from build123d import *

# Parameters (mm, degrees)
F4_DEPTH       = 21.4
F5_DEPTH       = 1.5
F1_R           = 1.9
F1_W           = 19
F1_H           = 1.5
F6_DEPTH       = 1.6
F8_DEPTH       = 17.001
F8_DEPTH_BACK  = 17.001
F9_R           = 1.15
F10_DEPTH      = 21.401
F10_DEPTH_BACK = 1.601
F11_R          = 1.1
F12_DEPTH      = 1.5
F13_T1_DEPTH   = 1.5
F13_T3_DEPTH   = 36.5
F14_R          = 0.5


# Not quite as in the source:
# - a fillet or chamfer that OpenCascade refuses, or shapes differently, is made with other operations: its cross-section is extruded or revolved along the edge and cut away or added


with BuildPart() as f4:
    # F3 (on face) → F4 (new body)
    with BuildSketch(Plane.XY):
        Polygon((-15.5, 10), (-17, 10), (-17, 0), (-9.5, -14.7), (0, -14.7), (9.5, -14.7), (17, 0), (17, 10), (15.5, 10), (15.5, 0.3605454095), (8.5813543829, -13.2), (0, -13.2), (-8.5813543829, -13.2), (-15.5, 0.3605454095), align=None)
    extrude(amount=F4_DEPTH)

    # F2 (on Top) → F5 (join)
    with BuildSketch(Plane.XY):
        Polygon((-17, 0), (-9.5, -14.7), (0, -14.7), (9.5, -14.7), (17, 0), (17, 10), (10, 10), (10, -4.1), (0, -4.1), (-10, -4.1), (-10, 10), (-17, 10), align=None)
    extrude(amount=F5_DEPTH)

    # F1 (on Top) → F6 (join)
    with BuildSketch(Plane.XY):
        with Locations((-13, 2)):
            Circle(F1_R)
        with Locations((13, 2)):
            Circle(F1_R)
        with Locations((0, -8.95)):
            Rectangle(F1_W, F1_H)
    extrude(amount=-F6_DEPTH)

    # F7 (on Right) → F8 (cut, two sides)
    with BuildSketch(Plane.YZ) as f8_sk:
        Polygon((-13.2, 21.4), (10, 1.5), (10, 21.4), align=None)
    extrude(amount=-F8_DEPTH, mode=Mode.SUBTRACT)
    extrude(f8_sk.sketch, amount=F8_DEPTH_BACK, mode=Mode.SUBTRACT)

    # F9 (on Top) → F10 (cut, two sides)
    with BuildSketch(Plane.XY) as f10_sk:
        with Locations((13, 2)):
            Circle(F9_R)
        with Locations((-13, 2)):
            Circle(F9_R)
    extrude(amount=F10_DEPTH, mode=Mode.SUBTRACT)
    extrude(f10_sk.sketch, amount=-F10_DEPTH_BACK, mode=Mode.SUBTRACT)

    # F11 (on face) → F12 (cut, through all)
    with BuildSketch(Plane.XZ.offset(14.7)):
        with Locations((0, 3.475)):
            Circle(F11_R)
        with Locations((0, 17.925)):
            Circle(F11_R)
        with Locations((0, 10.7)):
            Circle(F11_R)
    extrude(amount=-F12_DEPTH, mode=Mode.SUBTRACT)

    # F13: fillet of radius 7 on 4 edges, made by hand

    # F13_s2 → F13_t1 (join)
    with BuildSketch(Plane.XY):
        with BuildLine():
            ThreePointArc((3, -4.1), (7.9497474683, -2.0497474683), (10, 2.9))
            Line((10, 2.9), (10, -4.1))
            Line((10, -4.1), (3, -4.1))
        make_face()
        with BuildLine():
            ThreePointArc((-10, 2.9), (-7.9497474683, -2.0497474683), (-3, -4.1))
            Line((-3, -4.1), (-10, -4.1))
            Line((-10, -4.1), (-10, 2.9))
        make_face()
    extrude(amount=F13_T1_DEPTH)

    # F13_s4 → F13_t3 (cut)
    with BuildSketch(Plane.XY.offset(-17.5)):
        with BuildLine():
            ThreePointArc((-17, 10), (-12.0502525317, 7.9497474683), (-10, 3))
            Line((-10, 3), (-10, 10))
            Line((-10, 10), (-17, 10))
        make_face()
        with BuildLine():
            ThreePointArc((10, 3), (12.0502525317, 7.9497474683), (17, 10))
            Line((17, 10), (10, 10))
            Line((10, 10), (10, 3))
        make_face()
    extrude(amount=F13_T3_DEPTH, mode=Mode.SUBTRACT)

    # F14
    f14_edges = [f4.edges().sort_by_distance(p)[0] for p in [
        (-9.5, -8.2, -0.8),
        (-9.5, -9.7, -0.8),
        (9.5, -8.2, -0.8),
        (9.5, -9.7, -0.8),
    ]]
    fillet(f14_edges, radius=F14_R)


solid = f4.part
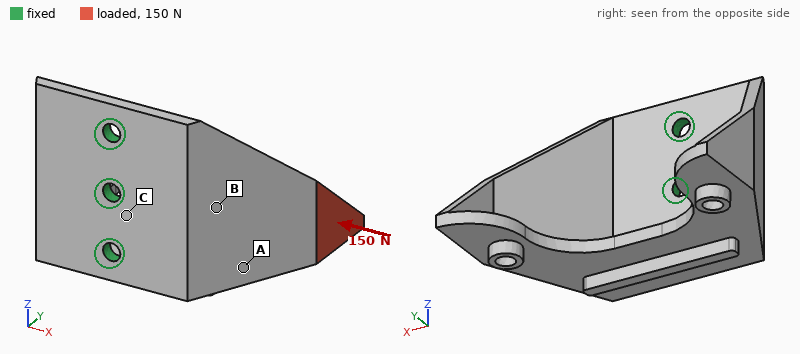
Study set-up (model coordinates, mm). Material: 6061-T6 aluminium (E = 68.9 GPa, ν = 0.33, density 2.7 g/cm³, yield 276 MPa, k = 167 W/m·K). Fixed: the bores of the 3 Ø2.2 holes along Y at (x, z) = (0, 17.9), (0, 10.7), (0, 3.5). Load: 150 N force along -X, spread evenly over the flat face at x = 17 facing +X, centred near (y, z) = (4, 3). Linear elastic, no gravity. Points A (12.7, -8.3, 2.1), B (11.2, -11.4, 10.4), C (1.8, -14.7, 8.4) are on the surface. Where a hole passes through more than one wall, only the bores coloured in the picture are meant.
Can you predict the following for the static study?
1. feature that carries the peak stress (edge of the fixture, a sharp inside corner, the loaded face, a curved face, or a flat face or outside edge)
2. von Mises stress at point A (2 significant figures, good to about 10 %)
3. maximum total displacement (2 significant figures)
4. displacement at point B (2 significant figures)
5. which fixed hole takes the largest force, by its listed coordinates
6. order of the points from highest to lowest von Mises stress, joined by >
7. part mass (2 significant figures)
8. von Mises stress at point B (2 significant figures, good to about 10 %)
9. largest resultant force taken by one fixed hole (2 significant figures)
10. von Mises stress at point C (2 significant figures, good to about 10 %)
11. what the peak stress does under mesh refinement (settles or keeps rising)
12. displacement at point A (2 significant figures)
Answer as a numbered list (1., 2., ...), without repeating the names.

1. edge of the fixture
2. 50 MPa
3. 0.38 mm
4. 0.092 mm
5. (0, 3.5)
6. C > A > B
7. 5.6 g
8. 29 MPa
9. 140 N
10. 92 MPa
11. keeps rising
12. 0.15 mm
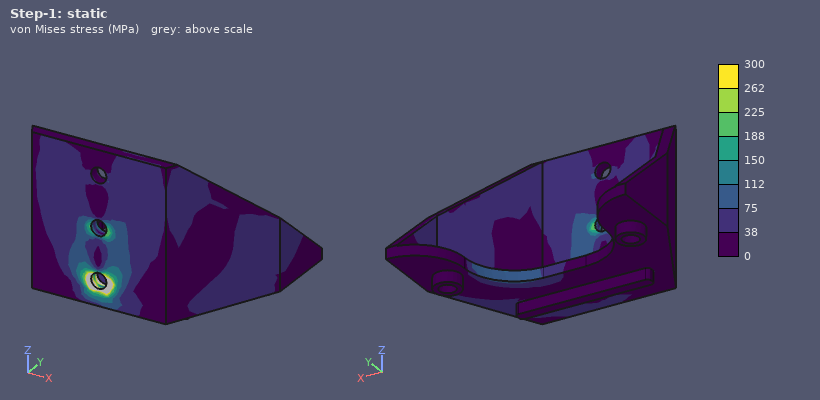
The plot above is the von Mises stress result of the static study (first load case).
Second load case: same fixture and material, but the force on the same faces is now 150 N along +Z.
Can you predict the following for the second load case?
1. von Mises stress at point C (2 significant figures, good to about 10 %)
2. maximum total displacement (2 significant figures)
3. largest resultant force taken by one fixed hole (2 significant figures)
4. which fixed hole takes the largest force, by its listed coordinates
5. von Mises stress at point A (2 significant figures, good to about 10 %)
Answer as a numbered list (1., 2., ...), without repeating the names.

1. 31 MPa
2. 0.27 mm
3. 250 N
4. (0, 3.5)
5. 44 MPa
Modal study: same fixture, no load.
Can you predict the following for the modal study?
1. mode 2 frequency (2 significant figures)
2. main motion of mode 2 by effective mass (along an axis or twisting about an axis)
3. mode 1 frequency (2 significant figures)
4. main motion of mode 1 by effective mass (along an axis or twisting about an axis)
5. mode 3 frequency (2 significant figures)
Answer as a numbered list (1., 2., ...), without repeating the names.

1. 4700 Hz
2. along Z
3. 2600 Hz
4. along X
5. 5300 Hz
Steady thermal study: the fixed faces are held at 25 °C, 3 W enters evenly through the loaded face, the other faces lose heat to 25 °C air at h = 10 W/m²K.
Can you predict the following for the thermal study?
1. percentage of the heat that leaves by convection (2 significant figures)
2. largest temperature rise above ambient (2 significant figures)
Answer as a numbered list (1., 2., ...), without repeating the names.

1. 3.3 %
2. 16 K
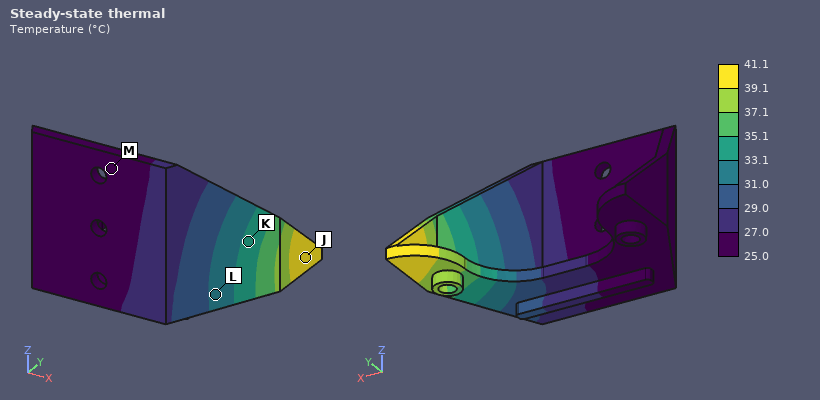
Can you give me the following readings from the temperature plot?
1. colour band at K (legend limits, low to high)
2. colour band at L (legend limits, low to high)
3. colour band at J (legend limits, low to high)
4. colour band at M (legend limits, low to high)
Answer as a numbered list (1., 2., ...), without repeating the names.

1. 33.1 to 35.1 °C
2. 31.0 to 33.1 °C
3. 39.1 to 41.1 °C
4. 25.0 to 27.0 °C
